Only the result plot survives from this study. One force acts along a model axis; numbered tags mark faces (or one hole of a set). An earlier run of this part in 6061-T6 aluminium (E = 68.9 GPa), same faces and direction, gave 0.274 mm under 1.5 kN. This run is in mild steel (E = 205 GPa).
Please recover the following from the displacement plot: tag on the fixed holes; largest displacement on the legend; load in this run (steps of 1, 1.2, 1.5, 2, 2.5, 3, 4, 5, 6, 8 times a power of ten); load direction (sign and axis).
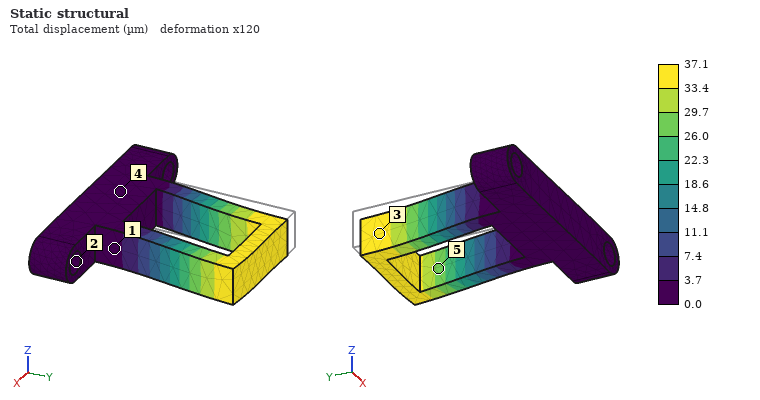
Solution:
2
37.1 µm
600 N
+X
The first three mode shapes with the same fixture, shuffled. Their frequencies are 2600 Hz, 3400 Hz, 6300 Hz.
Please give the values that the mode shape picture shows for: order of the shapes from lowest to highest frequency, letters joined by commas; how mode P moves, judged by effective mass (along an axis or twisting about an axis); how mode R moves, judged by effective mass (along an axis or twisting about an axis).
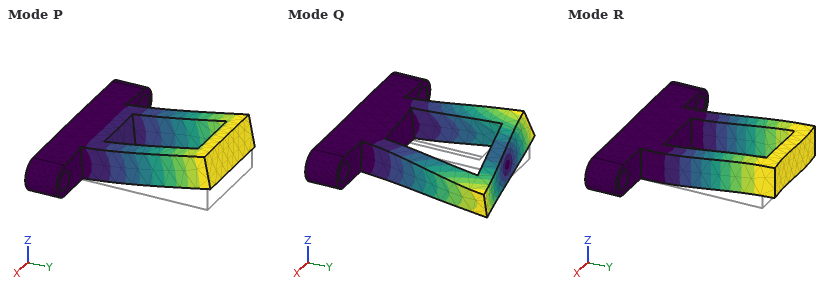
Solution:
P, R, Q
along Z
along X
